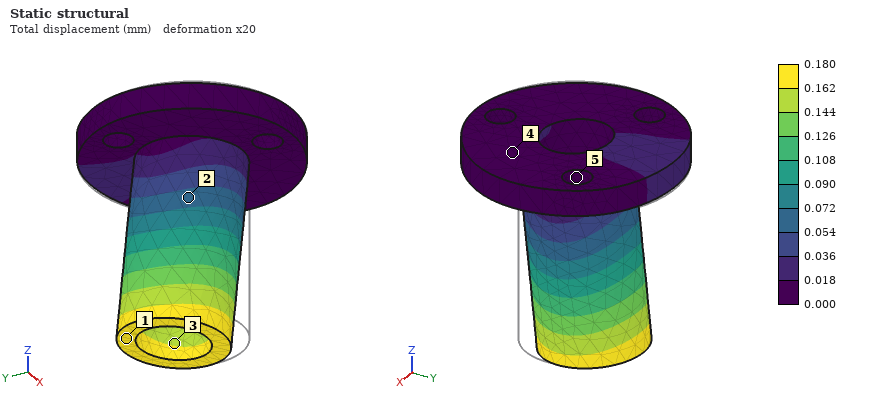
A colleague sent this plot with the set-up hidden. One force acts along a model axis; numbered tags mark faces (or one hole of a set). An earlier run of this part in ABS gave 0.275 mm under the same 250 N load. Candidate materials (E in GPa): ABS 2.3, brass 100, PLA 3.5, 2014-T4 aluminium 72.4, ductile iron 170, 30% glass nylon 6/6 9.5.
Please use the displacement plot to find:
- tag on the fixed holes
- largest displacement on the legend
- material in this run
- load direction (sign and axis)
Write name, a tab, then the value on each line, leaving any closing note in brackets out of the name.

tag on the fixed holes	5
largest displacement on the legend	0.180 mm
material in this run	PLA
load direction	+Y
